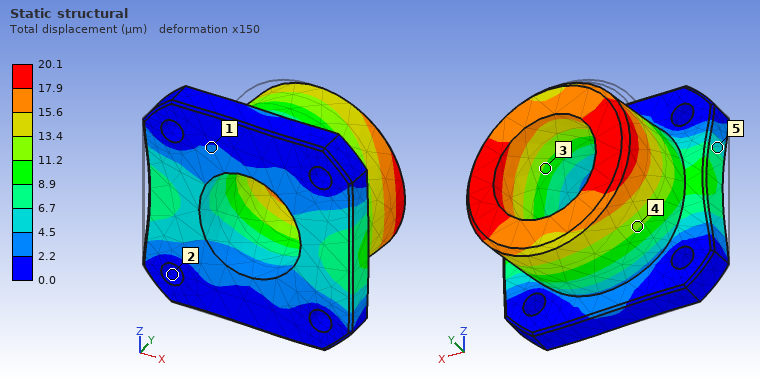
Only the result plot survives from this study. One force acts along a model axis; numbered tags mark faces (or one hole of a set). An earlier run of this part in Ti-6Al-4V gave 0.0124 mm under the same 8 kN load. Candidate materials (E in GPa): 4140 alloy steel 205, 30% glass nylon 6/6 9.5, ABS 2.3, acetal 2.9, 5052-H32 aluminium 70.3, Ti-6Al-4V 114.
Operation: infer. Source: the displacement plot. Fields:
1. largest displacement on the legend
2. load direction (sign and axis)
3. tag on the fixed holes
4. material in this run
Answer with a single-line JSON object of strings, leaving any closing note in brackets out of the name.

{"largest displacement on the legend": "20.1 µm", "load direction": "+X", "tag on the fixed holes": "2", "material in this run": "5052-H32 aluminium"}
